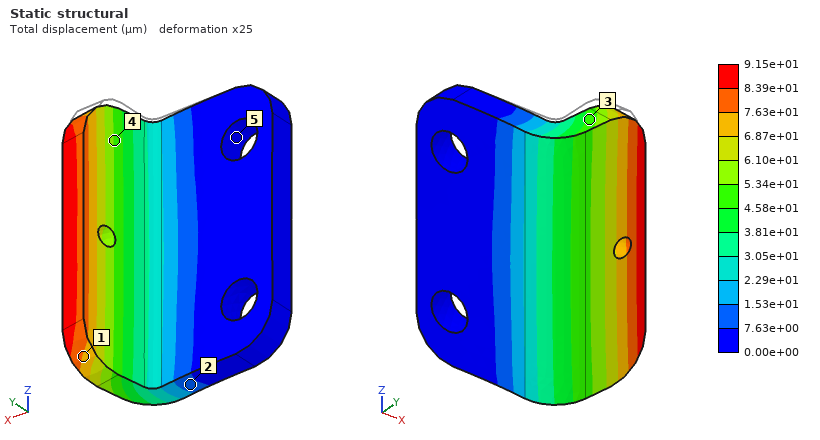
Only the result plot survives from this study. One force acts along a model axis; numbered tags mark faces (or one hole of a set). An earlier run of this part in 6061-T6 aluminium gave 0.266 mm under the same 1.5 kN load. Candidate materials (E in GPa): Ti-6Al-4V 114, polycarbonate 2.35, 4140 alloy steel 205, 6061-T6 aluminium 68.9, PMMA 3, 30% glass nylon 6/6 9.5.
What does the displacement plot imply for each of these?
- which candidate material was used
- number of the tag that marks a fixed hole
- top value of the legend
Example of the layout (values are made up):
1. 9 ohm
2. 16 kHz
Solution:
1. 4140 alloy steel
2. 5
3. 9.15e+01 µm
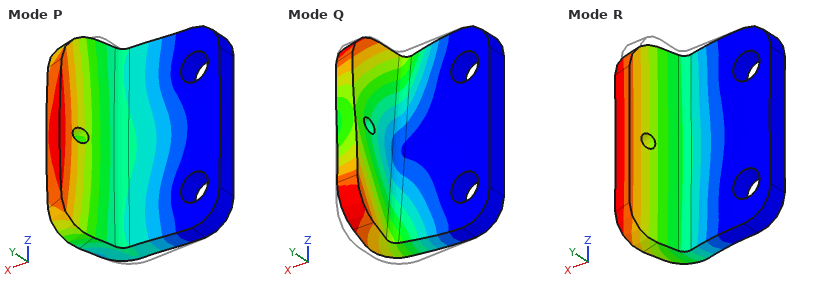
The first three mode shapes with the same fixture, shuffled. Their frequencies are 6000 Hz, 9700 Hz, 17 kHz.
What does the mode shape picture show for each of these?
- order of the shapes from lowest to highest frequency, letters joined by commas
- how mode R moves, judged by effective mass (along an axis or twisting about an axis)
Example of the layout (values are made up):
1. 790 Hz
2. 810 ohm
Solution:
1. R, Q, P
2. along Y
